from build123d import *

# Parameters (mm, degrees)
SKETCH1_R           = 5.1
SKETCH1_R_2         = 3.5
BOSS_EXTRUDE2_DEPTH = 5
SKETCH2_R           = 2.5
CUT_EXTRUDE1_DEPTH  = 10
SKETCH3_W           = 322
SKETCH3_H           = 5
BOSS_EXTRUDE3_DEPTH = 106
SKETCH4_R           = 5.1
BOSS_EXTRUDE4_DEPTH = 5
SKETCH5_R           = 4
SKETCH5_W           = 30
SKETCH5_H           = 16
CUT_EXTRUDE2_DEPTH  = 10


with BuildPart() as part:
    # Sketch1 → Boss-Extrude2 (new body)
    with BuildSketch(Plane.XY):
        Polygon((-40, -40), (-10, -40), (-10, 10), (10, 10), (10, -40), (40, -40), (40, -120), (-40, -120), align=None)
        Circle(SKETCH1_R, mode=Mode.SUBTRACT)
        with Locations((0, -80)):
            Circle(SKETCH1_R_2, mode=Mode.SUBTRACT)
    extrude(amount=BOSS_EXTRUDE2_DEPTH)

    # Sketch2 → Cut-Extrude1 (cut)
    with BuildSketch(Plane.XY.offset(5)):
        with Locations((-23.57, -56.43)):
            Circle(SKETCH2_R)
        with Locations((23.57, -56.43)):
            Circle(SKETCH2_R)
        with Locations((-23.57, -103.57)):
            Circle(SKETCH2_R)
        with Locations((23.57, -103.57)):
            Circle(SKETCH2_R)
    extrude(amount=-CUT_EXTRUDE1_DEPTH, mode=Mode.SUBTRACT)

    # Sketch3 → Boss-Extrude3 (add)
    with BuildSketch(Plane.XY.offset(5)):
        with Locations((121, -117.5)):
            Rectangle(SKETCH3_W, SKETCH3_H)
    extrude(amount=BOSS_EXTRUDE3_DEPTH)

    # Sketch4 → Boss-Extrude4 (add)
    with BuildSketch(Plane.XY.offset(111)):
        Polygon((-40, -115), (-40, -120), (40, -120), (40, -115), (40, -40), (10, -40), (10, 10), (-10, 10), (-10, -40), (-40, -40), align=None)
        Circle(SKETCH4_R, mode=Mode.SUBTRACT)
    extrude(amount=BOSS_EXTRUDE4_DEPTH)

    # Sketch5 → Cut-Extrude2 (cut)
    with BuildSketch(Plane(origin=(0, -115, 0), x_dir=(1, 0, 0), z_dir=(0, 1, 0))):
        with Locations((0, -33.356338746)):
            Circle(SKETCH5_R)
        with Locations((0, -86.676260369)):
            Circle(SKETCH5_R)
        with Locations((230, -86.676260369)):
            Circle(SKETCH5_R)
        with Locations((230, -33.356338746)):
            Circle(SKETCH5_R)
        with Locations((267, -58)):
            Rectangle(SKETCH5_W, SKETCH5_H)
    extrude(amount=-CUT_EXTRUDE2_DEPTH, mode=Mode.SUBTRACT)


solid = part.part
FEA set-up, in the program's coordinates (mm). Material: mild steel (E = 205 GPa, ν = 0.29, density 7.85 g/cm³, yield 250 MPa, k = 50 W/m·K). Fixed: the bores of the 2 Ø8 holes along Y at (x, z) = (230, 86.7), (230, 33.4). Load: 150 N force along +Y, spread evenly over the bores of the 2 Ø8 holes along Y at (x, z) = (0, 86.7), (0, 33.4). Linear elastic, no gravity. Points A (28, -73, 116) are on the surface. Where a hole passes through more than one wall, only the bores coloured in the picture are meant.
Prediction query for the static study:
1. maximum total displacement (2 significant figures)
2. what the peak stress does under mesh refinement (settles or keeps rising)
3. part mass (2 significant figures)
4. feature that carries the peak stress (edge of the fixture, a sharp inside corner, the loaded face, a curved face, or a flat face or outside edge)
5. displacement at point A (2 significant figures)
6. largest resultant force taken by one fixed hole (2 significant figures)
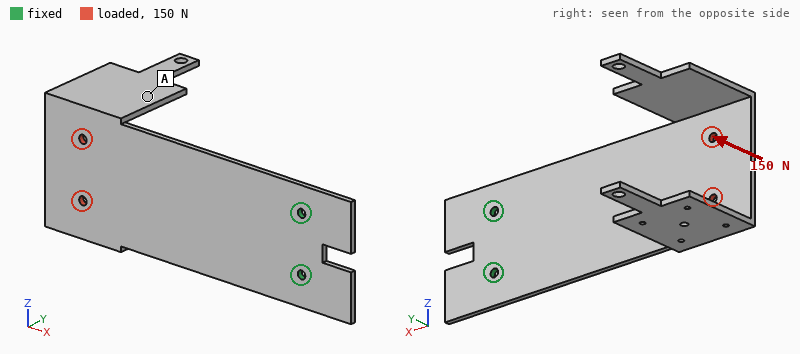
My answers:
3.6 mm
keeps rising
1.9 kg
edge of the fixture
2.3 mm
77 N
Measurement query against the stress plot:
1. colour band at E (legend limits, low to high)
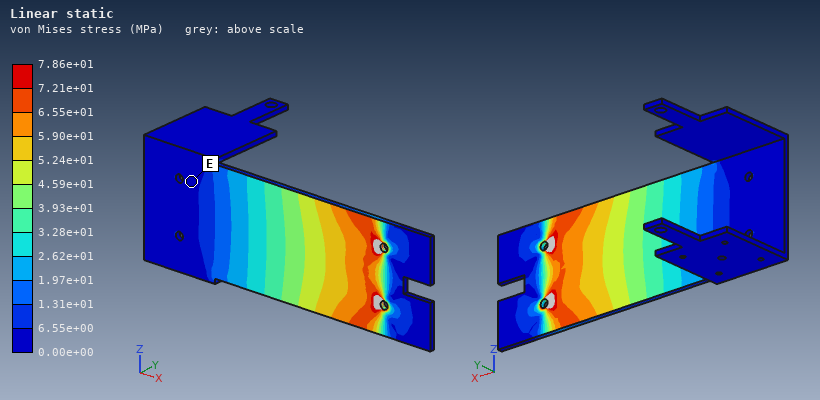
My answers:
0.00e+00 to 6.55e+00 MPa
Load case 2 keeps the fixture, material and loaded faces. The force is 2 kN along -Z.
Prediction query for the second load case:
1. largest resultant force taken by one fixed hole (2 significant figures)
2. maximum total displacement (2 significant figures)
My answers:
8.1 kN
0.15 mm
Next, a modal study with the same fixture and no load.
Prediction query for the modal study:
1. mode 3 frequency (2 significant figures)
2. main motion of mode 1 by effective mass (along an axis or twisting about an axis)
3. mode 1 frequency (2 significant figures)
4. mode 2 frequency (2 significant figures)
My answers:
220 Hz
along Y
36 Hz
110 Hz
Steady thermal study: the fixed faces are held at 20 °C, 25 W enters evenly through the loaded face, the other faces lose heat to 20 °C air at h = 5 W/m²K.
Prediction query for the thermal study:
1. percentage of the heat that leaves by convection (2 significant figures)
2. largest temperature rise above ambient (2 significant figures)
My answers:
78 %
80 K
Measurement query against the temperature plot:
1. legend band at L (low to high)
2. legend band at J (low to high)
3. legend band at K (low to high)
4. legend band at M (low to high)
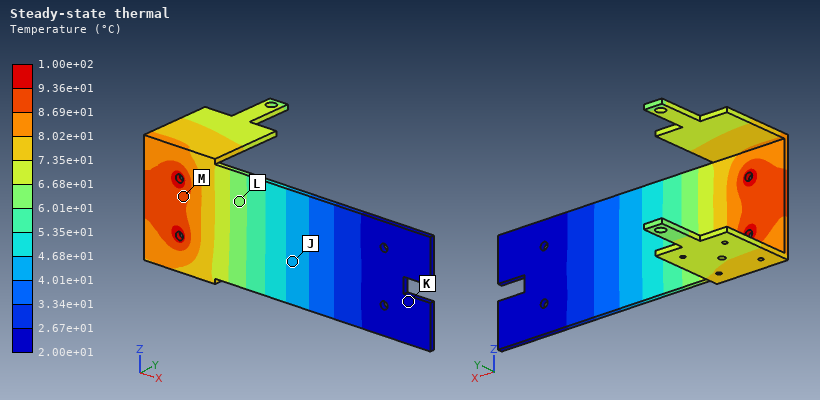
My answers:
6.01e+01 to 6.68e+01 °C
4.01e+01 to 4.68e+01 °C
2.00e+01 to 2.67e+01 °C
8.69e+01 to 9.36e+01 °C
